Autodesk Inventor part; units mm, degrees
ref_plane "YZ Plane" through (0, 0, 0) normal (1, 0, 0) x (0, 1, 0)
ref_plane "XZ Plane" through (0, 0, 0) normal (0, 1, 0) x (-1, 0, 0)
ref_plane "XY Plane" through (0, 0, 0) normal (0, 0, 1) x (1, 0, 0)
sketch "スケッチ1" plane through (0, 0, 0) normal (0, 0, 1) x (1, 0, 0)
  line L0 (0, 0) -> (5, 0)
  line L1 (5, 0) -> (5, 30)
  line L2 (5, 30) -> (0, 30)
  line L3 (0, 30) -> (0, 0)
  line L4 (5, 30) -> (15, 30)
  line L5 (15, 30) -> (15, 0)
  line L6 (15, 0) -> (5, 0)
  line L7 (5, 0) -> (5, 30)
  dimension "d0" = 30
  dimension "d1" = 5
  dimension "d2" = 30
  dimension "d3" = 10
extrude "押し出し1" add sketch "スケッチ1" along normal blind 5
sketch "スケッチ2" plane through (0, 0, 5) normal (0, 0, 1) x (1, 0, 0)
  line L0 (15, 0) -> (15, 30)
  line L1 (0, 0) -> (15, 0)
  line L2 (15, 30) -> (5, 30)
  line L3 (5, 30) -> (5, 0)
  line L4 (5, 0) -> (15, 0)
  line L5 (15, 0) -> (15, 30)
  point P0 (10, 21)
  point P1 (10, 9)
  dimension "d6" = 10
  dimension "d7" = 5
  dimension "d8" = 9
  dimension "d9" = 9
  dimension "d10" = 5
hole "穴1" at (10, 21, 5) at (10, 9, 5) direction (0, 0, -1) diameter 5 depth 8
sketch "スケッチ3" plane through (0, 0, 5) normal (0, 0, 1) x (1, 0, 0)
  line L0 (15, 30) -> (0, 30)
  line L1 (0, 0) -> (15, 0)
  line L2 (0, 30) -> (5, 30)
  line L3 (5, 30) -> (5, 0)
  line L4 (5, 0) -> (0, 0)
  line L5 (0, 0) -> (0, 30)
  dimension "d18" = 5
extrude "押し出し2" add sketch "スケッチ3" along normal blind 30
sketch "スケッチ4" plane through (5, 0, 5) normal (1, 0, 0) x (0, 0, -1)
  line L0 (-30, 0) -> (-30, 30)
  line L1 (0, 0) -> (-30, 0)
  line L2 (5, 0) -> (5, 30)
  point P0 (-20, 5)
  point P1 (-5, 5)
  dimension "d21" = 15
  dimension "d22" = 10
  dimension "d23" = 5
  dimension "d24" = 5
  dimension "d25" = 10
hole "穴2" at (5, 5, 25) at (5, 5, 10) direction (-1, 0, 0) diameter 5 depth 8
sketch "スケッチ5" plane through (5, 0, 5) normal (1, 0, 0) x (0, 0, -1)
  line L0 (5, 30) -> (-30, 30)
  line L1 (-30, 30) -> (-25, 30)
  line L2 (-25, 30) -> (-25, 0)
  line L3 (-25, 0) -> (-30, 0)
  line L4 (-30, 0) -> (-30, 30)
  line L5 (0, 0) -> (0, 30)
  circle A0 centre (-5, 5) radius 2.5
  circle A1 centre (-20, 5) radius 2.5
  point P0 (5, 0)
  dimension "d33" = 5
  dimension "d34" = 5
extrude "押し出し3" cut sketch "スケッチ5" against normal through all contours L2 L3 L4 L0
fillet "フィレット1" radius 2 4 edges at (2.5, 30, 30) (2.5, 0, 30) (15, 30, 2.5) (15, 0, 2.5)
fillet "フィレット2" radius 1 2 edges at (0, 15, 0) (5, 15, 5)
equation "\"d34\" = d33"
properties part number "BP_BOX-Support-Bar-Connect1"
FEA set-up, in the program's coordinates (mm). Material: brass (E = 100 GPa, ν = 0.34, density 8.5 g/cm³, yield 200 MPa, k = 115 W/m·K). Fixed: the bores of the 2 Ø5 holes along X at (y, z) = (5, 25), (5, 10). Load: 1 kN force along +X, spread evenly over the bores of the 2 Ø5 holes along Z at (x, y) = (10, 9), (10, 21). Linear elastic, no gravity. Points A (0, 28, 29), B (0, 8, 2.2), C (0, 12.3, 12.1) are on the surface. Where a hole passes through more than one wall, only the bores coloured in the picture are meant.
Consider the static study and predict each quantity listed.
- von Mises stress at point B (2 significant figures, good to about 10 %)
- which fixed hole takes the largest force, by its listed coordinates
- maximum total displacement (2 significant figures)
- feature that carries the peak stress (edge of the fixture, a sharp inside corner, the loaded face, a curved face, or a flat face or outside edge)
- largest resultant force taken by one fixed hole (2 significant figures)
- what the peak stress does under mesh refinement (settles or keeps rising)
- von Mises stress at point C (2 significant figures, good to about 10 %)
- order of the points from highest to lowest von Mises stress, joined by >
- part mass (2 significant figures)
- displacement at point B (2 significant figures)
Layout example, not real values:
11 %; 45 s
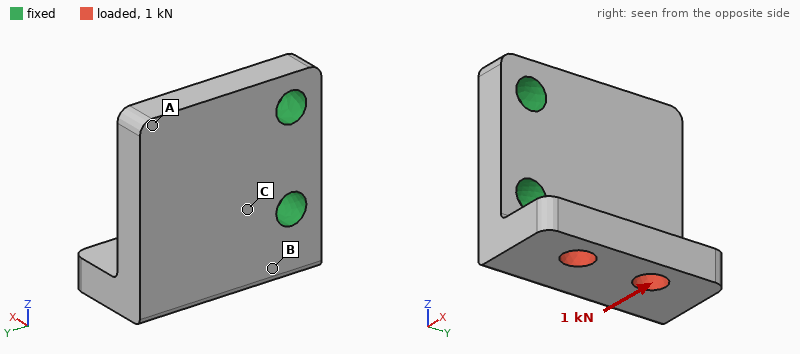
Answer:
31 MPa; (5, 10); 66 µm; edge of the fixture; 1.1 kN; keeps rising; 49 MPa; C > B > A; 48 g; 13 µm
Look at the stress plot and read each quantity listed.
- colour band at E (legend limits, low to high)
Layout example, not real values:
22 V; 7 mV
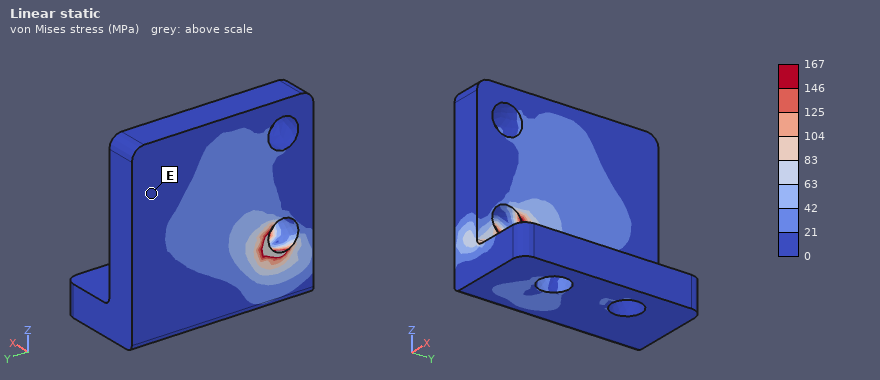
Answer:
0 to 21 MPa
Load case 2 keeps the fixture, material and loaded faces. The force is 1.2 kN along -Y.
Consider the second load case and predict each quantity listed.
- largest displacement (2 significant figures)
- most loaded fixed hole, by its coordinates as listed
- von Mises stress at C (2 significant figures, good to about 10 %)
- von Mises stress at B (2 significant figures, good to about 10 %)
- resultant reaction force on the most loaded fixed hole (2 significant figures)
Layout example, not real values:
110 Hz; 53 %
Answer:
54 µm; (5, 10); 33 MPa; 21 MPa; 1.5 kN
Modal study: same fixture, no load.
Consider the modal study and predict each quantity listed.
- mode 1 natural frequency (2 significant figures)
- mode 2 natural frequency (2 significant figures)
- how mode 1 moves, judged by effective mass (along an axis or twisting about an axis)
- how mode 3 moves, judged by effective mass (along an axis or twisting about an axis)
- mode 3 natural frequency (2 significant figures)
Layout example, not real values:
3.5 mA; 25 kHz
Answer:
4400 Hz; 6800 Hz; along X; along Z; 10 kHz
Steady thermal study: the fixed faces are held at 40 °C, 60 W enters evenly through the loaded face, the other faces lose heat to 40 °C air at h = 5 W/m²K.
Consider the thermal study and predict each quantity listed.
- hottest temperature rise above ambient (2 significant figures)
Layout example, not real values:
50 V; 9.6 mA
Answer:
79 K
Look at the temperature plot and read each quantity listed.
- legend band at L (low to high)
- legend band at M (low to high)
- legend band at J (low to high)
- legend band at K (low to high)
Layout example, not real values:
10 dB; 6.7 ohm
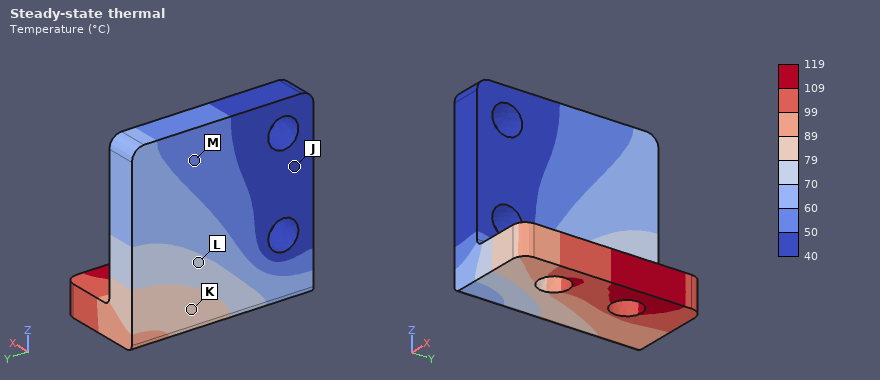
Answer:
70 to 79 °C; 50 to 60 °C; 40 to 50 °C; 79 to 89 °C
